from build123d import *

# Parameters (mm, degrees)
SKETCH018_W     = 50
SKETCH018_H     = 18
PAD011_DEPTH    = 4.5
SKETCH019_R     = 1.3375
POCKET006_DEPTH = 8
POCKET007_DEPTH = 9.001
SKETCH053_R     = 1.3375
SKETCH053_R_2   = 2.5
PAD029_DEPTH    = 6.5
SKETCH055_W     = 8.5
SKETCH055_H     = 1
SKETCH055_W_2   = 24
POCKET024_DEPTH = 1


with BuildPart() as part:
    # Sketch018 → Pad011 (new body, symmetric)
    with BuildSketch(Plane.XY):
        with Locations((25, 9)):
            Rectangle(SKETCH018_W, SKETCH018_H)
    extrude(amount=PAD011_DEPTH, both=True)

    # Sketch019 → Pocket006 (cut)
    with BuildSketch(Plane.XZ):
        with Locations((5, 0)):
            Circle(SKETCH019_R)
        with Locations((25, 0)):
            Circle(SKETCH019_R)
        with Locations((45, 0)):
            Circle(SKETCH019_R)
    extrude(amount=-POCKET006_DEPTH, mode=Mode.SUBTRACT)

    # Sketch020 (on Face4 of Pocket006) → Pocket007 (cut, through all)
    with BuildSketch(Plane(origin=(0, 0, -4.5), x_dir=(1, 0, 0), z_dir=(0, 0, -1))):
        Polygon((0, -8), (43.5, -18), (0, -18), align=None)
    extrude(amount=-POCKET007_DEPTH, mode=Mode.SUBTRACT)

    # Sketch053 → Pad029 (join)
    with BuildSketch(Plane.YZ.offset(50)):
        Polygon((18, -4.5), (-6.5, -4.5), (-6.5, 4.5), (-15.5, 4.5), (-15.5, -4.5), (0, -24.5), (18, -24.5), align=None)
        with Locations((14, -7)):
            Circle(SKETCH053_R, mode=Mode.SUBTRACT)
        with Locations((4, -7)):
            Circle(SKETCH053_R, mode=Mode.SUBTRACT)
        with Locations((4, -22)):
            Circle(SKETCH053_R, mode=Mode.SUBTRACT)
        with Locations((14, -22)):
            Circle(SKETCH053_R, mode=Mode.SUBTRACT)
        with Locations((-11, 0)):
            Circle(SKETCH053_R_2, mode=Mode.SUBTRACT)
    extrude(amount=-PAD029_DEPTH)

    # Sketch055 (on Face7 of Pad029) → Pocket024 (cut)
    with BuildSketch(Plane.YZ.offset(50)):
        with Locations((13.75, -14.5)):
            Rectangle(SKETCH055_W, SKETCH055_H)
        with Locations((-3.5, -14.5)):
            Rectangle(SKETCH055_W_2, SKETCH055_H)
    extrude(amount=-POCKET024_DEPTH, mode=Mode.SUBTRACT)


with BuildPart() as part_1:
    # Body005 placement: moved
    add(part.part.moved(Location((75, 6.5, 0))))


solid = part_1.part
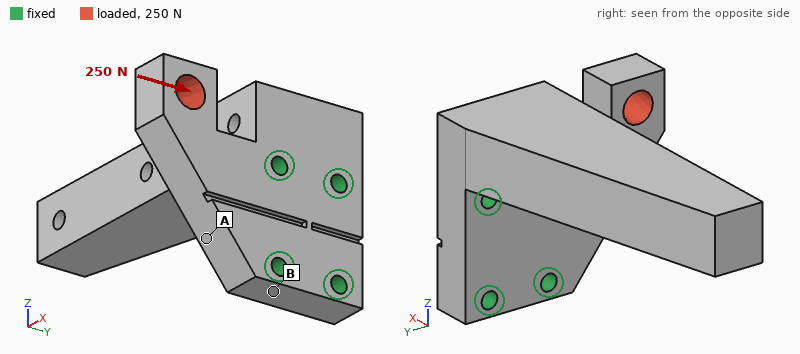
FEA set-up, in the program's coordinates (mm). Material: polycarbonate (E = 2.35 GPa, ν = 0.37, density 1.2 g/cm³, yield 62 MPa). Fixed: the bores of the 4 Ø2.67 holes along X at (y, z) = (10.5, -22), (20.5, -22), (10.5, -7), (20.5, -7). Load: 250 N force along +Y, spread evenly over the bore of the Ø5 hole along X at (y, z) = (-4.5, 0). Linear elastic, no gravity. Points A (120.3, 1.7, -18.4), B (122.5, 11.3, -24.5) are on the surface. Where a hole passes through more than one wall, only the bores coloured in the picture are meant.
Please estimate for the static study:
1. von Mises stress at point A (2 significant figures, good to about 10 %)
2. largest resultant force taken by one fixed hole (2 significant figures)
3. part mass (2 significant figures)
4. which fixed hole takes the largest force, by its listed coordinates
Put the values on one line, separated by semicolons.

7.2 MPa; 320 N; 11 g; (10.5, -7)
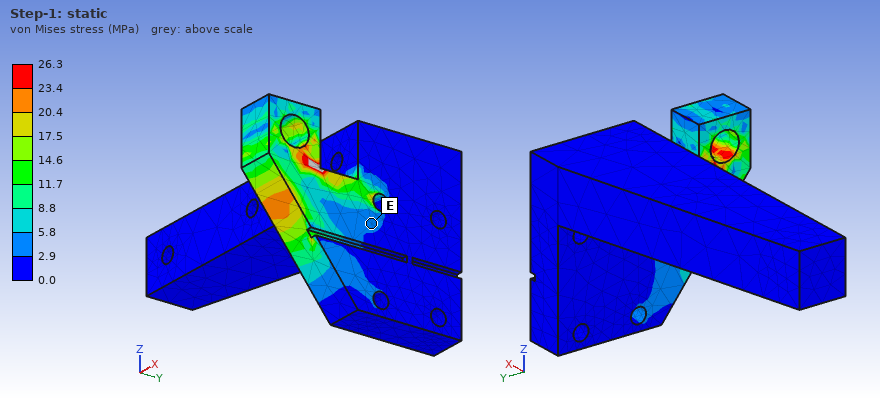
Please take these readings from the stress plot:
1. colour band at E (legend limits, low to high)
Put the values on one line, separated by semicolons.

2.9 to 5.8 MPa
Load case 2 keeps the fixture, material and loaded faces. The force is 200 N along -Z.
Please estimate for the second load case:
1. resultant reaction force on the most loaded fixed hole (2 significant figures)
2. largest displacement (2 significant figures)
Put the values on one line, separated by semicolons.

190 N; 0.23 mm
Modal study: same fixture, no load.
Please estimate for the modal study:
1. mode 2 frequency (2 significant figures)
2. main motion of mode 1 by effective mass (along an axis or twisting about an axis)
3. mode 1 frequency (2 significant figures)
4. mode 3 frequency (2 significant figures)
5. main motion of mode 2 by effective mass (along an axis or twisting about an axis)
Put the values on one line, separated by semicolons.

1400 Hz; along Z; 820 Hz; 3200 Hz; along Y
